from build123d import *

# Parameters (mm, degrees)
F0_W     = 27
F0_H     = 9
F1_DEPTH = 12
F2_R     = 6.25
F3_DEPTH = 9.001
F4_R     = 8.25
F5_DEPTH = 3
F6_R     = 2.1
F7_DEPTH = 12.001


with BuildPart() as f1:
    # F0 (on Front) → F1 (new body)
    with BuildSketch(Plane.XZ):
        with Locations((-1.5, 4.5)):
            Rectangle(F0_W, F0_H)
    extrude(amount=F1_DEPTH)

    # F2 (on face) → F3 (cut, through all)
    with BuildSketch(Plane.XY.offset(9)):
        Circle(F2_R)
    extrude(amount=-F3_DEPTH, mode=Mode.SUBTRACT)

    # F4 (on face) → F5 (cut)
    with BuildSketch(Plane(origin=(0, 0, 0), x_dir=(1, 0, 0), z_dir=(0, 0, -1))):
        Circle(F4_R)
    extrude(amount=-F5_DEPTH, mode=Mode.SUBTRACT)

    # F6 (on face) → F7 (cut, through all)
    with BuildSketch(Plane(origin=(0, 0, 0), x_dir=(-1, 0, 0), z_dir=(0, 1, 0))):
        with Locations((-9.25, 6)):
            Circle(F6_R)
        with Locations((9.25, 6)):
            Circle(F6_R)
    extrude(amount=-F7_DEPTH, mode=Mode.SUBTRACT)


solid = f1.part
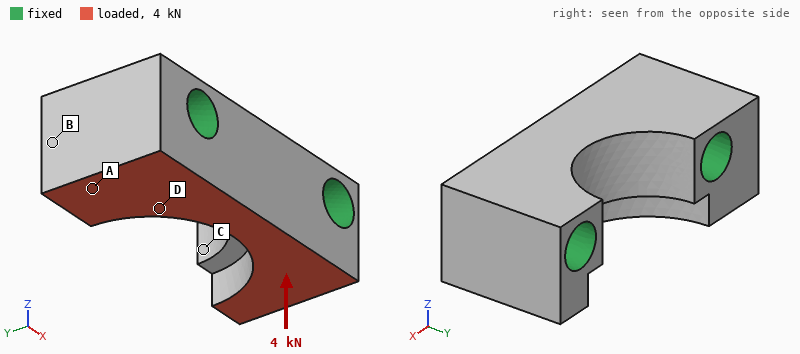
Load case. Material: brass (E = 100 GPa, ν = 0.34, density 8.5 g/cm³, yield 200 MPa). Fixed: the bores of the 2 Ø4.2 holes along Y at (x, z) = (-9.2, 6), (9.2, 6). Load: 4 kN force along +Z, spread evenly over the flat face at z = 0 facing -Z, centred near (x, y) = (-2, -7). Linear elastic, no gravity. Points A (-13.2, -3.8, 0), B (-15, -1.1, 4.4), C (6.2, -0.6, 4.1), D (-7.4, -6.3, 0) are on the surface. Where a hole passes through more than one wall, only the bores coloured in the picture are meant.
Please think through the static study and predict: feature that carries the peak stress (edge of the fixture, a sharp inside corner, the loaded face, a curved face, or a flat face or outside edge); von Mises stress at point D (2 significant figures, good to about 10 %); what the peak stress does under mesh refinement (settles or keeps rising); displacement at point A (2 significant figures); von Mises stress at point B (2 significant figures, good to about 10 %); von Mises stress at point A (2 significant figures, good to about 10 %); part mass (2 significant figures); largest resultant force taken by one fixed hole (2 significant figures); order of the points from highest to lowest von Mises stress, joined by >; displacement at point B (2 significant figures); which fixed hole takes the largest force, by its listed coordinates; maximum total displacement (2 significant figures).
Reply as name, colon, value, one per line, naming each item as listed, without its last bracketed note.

feature that carries the peak stress: edge of the fixture
von Mises stress at point D: 29 MPa
what the peak stress does under mesh refinement: keeps rising
displacement at point A: 1.9 µm
von Mises stress at point B: 11 MPa
von Mises stress at point A: 19 MPa
part mass: 16 g
largest resultant force taken by one fixed hole: 2.4 kN
order of the points from highest to lowest von Mises stress, joined by >: D > A > B > C
displacement at point B: 1.3 µm
which fixed hole takes the largest force, by its listed coordinates: (-9.2, 6)
maximum total displacement: 3.4 µm
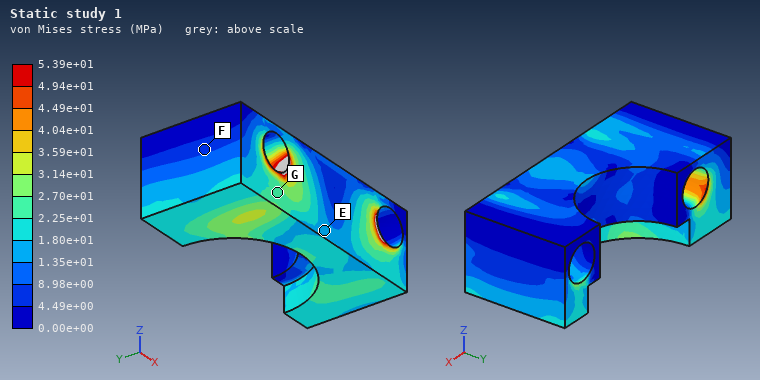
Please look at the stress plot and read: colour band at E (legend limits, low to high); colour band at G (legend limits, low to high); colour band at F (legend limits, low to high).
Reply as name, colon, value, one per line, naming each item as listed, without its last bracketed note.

colour band at E: 1.35e+01 to 1.80e+01 MPa
colour band at G: 2.25e+01 to 2.70e+01 MPa
colour band at F: 4.49e+00 to 8.98e+00 MPa
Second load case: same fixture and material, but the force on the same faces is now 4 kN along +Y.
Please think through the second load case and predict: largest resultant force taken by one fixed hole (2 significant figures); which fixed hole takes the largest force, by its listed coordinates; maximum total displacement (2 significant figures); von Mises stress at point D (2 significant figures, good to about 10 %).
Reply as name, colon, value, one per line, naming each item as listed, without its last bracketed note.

largest resultant force taken by one fixed hole: 2.3 kN
which fixed hole takes the largest force, by its listed coordinates: (-9.2, 6)
maximum total displacement: 9.5 µm
von Mises stress at point D: 42 MPa
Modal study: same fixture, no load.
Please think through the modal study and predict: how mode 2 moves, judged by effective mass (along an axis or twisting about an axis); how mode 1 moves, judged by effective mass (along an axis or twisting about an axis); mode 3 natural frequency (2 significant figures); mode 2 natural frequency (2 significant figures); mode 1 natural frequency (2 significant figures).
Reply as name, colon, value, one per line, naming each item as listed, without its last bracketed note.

how mode 2 moves, judged by effective mass: along Y
how mode 1 moves, judged by effective mass: along Z
mode 3 natural frequency: 68 kHz
mode 2 natural frequency: 61 kHz
mode 1 natural frequency: 51 kHz
